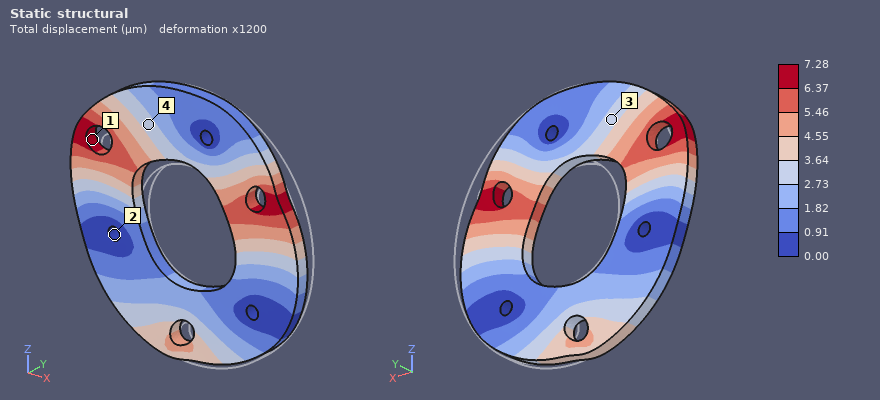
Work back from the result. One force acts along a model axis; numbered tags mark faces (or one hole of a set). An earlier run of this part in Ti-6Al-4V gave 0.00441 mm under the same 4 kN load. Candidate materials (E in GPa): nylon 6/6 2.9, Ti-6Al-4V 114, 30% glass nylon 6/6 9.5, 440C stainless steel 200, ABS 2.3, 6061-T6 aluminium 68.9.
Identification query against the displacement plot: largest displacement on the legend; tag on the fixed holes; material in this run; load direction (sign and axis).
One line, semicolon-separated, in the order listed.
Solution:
7.28 µm; 2; 6061-T6 aluminium; -X
